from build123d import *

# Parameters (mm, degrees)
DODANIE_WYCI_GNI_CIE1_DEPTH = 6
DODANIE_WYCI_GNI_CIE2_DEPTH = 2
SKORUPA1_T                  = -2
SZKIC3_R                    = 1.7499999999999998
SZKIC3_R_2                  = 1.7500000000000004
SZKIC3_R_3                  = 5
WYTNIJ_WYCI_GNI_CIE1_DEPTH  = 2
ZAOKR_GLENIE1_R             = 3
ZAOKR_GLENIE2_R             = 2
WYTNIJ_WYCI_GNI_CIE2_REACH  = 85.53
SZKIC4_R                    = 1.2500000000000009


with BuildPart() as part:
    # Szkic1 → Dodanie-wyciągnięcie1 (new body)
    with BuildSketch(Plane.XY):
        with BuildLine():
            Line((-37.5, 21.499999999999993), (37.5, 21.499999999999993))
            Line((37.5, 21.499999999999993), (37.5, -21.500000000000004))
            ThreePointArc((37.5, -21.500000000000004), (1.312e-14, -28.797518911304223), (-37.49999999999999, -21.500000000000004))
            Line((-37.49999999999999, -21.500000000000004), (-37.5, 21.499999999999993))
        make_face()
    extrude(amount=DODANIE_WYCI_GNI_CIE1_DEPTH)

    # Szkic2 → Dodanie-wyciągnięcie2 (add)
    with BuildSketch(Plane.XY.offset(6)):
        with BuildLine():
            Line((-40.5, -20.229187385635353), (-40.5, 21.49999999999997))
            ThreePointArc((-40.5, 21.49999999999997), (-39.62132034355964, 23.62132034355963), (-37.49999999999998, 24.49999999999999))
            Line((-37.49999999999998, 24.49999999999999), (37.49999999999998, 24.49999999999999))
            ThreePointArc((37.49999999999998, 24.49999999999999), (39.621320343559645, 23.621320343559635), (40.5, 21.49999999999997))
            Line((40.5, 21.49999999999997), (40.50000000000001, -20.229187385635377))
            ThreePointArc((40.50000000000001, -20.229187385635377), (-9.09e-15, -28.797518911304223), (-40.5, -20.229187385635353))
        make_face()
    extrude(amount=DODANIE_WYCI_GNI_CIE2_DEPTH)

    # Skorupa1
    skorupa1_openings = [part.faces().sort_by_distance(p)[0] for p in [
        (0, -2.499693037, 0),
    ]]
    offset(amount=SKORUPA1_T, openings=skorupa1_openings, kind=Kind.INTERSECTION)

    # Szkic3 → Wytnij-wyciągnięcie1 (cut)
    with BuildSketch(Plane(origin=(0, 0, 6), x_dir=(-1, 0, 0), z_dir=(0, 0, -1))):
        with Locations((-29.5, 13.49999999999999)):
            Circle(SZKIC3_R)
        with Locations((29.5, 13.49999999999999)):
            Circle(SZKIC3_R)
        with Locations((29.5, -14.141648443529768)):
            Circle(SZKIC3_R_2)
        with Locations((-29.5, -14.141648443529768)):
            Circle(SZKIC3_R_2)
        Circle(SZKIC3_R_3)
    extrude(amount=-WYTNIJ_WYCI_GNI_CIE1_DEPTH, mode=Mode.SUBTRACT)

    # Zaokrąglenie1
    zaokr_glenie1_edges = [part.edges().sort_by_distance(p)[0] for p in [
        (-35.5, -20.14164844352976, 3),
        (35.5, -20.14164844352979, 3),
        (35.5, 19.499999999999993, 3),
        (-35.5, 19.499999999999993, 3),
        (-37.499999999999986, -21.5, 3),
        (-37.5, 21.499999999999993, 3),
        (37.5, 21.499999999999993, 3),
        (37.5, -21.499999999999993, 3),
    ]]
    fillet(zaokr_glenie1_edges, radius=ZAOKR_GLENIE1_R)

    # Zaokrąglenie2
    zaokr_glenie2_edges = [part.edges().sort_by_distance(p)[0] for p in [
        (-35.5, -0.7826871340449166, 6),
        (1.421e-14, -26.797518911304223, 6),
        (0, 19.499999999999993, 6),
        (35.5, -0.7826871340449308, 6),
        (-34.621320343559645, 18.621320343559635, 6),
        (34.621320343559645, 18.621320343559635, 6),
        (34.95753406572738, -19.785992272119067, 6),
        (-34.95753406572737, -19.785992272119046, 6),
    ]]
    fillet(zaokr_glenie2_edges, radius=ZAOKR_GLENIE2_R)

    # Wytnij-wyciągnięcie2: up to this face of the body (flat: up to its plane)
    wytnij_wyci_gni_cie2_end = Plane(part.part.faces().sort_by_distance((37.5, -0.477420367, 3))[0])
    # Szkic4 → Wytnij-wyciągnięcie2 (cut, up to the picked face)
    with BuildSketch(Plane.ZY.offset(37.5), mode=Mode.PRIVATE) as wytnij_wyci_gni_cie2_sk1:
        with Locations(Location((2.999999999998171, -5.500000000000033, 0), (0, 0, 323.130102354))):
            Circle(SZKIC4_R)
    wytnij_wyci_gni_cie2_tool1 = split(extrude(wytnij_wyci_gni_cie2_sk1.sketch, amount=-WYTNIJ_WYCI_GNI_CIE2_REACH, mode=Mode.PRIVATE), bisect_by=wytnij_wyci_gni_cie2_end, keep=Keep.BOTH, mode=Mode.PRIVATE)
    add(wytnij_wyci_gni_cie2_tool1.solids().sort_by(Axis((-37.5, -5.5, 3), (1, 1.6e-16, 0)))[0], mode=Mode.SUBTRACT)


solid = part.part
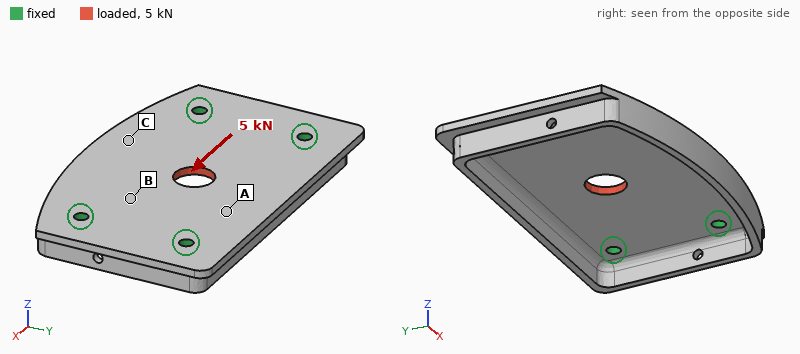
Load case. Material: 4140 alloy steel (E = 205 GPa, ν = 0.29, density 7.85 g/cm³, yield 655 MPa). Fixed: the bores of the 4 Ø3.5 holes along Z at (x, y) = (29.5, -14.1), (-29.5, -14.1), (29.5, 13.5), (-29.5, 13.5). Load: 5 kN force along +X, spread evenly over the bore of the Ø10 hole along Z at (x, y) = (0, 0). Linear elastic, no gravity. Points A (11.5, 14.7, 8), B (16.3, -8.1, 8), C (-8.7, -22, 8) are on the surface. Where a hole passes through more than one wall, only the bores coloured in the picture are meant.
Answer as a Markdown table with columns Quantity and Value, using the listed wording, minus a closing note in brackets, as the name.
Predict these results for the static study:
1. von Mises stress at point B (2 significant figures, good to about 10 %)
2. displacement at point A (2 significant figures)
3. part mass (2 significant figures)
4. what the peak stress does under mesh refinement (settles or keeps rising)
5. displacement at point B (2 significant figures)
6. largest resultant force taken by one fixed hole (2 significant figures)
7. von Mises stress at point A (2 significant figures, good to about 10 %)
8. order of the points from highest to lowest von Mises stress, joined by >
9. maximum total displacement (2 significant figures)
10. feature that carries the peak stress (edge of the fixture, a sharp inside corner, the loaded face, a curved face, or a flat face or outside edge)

| Quantity | Value |
|---|---|
| von Mises stress at point B | 42 MPa |
| displacement at point A | 2.9 µm |
| part mass | 85 g |
| what the peak stress does under mesh refinement | keeps rising |
| displacement at point B | 3.1 µm |
| largest resultant force taken by one fixed hole | 1.3 kN |
| von Mises stress at point A | 23 MPa |
| order of the points from highest to lowest von Mises stress, joined by > | B > A > C |
| maximum total displacement | 7.2 µm |
| feature that carries the peak stress | a sharp inside corner |
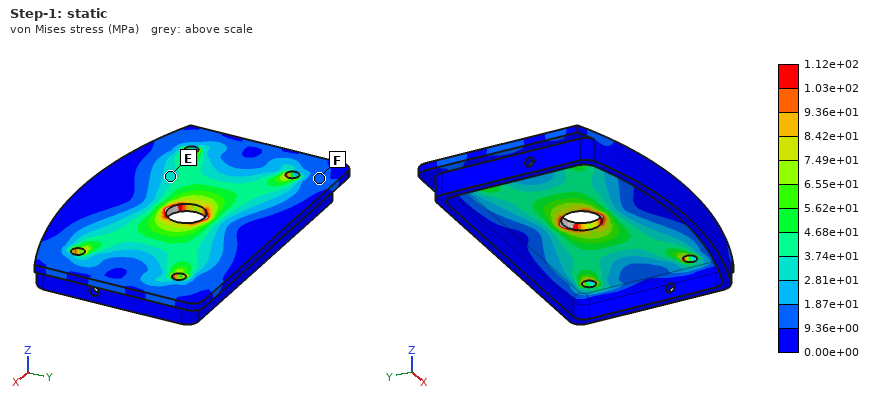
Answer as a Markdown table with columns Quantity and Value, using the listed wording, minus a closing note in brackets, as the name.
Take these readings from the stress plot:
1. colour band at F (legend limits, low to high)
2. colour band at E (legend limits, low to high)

| Quantity | Value |
|---|---|
| colour band at F | 9.36e+00 to 1.87e+01 MPa |
| colour band at E | 2.81e+01 to 3.74e+01 MPa |
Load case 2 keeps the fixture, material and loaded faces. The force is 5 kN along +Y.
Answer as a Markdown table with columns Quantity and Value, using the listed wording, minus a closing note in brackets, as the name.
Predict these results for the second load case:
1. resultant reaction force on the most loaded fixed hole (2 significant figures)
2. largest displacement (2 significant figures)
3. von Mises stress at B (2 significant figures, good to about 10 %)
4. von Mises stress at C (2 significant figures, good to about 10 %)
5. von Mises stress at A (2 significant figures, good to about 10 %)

| Quantity | Value |
|---|---|
| resultant reaction force on the most loaded fixed hole | 1.4 kN |
| largest displacement | 16 µm |
| von Mises stress at B | 47 MPa |
| von Mises stress at C | 33 MPa |
| von Mises stress at A | 41 MPa |
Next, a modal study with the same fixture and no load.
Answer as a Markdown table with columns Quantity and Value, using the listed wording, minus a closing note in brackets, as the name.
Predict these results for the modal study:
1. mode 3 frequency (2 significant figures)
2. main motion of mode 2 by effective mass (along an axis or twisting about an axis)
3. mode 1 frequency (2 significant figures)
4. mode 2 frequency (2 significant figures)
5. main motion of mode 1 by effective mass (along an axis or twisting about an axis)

| Quantity | Value |
|---|---|
| mode 3 frequency | 6000 Hz |
| main motion of mode 2 by effective mass | twisting about X |
| mode 1 frequency | 4100 Hz |
| mode 2 frequency | 4900 Hz |
| main motion of mode 1 by effective mass | along Z |
